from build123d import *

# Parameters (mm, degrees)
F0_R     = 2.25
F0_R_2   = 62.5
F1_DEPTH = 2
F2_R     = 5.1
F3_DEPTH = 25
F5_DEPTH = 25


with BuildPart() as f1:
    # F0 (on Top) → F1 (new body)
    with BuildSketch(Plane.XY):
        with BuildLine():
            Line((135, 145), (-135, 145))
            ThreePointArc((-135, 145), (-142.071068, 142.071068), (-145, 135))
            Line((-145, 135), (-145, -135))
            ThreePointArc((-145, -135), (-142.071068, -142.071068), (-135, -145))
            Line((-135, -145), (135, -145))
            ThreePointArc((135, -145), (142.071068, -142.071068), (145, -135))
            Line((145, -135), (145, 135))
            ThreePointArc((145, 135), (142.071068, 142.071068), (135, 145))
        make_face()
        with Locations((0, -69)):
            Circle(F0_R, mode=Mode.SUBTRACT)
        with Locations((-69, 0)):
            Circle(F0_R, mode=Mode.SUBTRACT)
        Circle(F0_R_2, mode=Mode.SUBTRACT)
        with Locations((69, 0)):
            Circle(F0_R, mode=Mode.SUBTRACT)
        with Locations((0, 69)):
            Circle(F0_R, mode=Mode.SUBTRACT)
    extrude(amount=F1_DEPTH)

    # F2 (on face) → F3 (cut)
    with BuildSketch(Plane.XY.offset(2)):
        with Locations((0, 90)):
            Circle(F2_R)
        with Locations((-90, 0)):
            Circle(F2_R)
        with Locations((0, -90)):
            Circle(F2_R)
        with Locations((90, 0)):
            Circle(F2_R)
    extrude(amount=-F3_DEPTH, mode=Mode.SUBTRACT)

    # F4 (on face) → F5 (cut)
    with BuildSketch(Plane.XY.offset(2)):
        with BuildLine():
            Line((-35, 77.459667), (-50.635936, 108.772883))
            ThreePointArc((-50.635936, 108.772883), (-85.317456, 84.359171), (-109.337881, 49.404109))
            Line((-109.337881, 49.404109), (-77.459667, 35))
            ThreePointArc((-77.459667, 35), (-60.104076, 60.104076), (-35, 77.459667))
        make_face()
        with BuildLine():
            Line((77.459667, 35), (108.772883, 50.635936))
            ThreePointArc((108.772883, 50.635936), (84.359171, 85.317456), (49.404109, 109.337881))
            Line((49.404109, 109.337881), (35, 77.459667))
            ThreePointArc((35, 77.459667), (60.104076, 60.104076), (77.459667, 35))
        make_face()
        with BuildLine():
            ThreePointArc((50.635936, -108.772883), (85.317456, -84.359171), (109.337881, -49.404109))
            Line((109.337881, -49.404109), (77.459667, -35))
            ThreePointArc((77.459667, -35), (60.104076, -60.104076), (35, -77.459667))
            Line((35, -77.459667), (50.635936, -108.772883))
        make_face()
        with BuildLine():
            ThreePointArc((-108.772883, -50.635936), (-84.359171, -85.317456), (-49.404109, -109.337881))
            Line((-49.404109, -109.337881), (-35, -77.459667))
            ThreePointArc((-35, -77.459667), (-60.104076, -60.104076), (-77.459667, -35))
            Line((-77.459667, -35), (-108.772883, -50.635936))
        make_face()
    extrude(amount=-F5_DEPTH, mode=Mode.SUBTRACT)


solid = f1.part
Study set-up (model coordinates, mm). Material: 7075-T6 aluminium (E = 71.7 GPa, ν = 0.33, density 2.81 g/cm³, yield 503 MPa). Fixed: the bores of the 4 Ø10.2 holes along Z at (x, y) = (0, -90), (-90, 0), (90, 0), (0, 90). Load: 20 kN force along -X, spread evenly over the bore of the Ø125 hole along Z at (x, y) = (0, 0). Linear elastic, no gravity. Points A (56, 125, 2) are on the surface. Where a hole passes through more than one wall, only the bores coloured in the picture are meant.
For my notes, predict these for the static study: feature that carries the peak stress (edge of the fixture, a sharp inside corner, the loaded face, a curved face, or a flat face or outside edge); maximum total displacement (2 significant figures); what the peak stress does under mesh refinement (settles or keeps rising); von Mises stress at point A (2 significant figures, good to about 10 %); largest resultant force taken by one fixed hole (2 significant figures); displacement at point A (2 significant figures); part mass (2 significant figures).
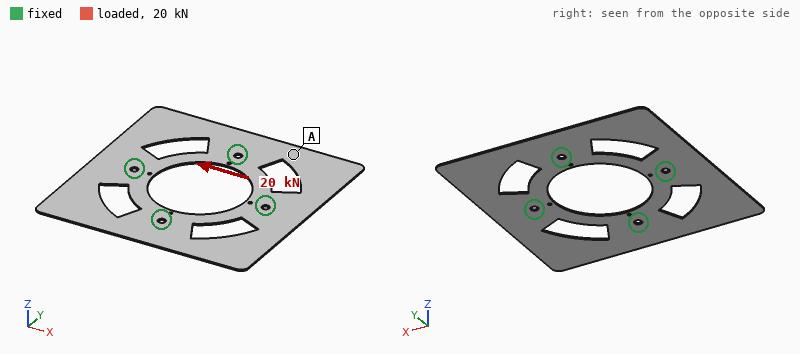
edge of the fixture
83 µm
keeps rising
13 MPa
5.5 kN
13 µm
340 g
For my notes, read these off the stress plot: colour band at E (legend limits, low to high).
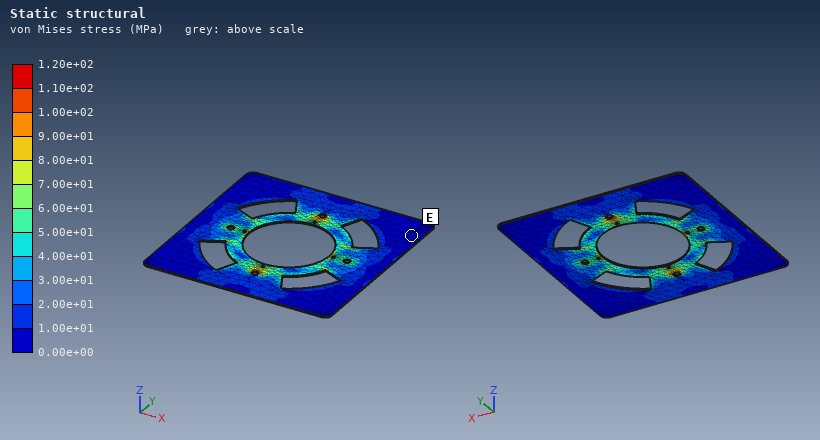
0.00e+00 to 1.00e+01 MPa
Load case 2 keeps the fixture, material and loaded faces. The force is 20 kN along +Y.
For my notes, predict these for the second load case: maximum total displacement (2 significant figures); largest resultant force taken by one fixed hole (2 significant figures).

83 µm
5.5 kN
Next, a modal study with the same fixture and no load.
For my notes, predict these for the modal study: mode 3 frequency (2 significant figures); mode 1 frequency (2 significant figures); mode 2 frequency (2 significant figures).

120 Hz
110 Hz
120 Hz
